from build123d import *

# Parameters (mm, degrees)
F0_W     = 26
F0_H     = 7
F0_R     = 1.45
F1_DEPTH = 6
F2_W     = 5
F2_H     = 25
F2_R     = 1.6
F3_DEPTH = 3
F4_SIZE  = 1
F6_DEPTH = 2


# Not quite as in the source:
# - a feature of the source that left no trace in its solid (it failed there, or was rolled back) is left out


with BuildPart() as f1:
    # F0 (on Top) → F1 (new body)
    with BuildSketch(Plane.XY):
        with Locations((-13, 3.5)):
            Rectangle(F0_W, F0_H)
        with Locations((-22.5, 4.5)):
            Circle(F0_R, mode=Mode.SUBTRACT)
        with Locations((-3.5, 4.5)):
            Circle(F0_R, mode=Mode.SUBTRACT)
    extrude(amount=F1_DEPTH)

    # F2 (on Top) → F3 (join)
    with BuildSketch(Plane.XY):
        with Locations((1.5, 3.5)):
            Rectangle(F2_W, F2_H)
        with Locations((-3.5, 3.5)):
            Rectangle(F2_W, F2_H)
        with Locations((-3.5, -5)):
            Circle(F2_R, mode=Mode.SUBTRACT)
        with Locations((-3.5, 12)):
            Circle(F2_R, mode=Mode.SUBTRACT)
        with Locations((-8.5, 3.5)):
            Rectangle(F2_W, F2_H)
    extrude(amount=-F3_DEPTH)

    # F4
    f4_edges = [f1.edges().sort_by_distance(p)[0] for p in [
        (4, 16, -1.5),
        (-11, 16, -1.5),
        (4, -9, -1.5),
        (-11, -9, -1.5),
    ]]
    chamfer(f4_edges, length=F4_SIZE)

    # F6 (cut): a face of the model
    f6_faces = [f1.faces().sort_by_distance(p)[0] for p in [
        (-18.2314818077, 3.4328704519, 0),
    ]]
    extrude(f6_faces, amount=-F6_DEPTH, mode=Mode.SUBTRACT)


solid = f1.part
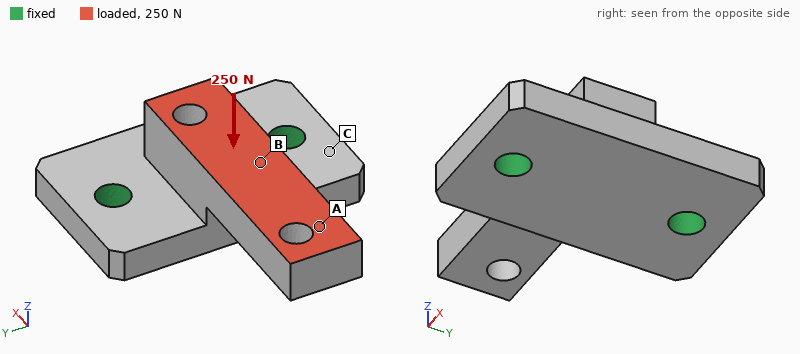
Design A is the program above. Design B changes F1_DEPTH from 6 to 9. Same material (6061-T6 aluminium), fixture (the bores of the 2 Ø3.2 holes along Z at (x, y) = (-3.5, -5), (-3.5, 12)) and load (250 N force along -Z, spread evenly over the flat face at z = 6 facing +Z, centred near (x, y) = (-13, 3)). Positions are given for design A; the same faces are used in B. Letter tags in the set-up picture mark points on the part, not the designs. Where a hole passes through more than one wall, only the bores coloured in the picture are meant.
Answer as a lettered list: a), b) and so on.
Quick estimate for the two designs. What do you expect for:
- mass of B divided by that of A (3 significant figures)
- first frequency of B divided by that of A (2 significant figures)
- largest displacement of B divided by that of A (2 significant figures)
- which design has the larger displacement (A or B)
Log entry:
a) 1.27
b) 0.85
c) 0.68
d) A
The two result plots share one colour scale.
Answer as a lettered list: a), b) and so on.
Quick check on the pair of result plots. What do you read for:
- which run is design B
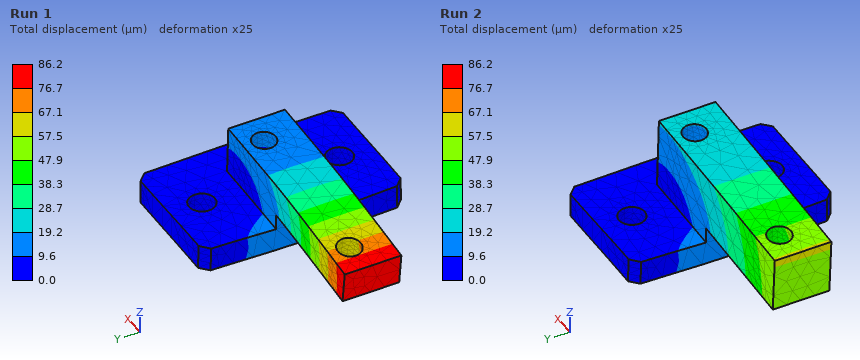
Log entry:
a) Run 2
